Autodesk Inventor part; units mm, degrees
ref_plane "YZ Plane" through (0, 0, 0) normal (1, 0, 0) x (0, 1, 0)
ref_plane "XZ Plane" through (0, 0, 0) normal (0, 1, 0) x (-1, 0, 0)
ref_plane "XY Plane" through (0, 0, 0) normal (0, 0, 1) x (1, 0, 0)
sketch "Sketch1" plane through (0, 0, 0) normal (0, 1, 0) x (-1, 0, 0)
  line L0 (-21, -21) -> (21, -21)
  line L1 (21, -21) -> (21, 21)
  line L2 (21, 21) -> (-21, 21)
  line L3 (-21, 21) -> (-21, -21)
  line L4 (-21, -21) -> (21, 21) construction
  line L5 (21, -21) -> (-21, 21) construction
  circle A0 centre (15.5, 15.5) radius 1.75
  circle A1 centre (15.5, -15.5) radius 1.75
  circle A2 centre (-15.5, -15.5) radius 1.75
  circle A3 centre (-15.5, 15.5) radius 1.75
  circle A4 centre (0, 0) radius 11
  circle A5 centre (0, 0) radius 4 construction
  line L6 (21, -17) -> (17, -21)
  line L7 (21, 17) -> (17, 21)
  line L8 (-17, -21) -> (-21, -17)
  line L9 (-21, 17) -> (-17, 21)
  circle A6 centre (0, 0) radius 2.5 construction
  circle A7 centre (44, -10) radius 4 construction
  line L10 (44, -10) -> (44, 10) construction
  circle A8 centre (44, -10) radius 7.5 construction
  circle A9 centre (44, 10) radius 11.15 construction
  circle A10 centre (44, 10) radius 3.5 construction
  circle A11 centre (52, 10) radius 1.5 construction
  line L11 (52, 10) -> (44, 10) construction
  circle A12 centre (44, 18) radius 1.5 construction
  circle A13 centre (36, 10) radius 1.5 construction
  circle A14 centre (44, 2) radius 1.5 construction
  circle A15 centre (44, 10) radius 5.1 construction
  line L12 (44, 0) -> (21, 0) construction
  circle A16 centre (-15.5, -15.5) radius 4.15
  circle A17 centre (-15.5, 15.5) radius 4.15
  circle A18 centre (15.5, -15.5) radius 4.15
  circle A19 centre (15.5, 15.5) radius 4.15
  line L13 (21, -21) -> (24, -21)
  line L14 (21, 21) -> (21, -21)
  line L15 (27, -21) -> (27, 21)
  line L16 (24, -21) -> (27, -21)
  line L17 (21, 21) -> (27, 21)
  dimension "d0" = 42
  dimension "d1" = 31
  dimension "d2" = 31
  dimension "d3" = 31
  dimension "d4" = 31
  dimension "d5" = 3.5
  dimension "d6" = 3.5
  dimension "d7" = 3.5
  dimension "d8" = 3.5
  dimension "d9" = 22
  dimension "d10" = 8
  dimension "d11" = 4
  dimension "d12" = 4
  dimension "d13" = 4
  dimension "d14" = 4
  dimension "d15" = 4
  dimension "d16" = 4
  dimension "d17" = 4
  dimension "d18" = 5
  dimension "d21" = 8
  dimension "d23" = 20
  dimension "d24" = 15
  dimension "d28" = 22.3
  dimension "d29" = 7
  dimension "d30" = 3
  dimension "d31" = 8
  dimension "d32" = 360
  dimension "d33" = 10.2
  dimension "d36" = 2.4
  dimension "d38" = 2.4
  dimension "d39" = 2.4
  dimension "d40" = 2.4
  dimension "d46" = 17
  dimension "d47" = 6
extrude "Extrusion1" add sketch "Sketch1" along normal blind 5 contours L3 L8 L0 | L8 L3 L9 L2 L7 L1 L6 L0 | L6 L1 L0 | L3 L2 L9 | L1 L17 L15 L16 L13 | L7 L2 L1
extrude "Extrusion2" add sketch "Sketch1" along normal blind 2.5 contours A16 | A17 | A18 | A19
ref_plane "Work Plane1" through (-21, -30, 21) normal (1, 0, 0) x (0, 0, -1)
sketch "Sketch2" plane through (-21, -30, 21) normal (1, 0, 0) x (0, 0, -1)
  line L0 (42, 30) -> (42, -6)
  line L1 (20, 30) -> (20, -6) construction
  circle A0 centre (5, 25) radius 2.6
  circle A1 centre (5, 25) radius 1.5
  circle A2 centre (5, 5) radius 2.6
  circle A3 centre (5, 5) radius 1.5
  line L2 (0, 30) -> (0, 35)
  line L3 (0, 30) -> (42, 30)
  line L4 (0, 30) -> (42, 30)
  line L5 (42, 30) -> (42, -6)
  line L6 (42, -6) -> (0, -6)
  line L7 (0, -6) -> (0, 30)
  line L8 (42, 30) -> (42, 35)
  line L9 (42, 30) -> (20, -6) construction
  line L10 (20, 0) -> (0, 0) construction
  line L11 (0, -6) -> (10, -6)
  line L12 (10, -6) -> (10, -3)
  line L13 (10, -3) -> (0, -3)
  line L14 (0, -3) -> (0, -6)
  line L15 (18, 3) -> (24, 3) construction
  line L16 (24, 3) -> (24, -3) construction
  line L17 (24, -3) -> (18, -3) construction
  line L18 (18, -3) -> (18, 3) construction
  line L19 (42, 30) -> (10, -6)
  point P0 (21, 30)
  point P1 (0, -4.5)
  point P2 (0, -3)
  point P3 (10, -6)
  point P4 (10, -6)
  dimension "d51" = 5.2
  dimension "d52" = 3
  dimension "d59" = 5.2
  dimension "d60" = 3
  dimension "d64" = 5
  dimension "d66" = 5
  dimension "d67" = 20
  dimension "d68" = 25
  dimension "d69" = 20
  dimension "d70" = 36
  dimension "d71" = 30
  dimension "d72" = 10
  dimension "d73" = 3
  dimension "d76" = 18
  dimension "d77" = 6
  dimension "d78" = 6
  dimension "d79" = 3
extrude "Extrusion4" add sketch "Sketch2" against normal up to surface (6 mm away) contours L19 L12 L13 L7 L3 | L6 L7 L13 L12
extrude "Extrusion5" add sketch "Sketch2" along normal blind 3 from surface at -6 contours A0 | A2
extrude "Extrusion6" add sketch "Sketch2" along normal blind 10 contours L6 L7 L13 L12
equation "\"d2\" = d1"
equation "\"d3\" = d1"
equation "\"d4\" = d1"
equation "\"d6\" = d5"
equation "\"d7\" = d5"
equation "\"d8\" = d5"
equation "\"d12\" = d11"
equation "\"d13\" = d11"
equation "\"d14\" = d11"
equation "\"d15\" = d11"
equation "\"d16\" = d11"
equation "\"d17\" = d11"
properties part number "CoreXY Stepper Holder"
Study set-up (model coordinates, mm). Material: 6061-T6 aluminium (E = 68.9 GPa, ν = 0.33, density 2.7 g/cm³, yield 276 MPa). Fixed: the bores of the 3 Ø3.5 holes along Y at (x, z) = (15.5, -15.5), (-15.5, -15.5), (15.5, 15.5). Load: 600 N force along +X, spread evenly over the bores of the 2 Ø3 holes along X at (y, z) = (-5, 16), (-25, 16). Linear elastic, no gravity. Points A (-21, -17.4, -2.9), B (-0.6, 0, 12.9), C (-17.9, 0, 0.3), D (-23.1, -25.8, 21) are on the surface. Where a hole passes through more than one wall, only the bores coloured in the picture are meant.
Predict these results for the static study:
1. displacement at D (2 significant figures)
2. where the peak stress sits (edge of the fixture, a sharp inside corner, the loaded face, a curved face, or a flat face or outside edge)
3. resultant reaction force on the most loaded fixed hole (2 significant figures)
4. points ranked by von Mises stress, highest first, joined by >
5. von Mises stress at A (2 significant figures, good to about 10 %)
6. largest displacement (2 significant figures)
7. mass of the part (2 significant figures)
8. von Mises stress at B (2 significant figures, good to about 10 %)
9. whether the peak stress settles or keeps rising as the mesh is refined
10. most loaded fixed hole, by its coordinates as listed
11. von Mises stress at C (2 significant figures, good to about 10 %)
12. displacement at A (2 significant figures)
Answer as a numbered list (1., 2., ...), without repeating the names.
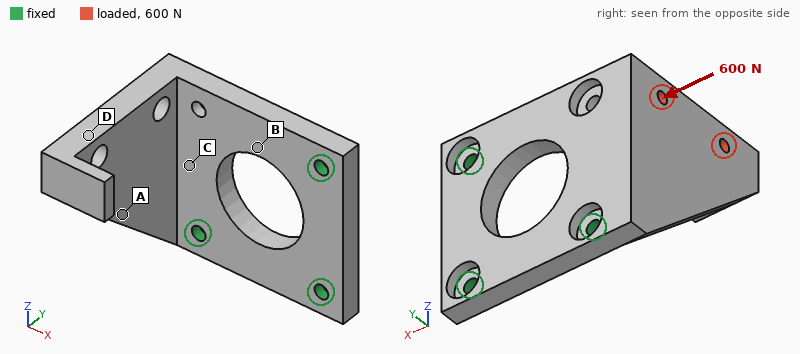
1. 0.39 mm
2. edge of the fixture
3. 560 N
4. B > C > A > D
5. 30 MPa
6. 0.53 mm
7. 36 g
8. 66 MPa
9. keeps rising
10. (15.5, 15.5)
11. 50 MPa
12. 0.20 mm
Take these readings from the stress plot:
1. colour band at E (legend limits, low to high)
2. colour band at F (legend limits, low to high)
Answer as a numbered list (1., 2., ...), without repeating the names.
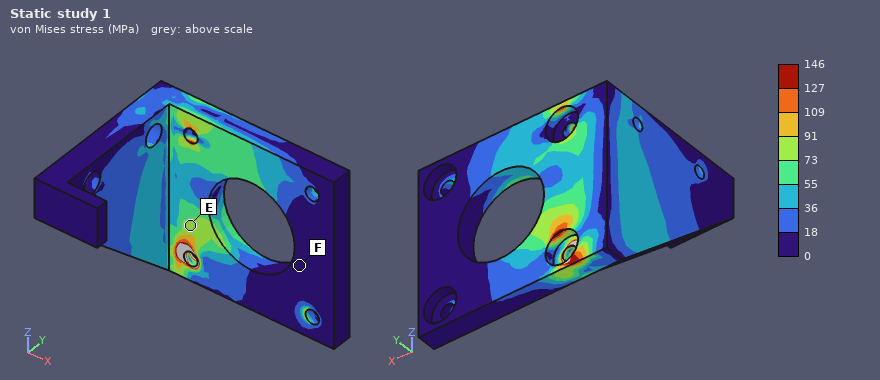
1. 73 to 91 MPa
2. 0 to 18 MPa
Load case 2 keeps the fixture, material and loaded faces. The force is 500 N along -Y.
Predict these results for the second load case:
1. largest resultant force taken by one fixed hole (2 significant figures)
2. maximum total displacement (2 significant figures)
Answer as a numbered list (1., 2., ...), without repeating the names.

1. 600 N
2. 0.59 mm
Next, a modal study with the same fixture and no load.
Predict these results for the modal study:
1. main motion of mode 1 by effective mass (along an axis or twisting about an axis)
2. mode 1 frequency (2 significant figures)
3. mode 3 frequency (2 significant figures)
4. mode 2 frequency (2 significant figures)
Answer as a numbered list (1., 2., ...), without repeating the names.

1. along Y
2. 1400 Hz
3. 7300 Hz
4. 2300 Hz
